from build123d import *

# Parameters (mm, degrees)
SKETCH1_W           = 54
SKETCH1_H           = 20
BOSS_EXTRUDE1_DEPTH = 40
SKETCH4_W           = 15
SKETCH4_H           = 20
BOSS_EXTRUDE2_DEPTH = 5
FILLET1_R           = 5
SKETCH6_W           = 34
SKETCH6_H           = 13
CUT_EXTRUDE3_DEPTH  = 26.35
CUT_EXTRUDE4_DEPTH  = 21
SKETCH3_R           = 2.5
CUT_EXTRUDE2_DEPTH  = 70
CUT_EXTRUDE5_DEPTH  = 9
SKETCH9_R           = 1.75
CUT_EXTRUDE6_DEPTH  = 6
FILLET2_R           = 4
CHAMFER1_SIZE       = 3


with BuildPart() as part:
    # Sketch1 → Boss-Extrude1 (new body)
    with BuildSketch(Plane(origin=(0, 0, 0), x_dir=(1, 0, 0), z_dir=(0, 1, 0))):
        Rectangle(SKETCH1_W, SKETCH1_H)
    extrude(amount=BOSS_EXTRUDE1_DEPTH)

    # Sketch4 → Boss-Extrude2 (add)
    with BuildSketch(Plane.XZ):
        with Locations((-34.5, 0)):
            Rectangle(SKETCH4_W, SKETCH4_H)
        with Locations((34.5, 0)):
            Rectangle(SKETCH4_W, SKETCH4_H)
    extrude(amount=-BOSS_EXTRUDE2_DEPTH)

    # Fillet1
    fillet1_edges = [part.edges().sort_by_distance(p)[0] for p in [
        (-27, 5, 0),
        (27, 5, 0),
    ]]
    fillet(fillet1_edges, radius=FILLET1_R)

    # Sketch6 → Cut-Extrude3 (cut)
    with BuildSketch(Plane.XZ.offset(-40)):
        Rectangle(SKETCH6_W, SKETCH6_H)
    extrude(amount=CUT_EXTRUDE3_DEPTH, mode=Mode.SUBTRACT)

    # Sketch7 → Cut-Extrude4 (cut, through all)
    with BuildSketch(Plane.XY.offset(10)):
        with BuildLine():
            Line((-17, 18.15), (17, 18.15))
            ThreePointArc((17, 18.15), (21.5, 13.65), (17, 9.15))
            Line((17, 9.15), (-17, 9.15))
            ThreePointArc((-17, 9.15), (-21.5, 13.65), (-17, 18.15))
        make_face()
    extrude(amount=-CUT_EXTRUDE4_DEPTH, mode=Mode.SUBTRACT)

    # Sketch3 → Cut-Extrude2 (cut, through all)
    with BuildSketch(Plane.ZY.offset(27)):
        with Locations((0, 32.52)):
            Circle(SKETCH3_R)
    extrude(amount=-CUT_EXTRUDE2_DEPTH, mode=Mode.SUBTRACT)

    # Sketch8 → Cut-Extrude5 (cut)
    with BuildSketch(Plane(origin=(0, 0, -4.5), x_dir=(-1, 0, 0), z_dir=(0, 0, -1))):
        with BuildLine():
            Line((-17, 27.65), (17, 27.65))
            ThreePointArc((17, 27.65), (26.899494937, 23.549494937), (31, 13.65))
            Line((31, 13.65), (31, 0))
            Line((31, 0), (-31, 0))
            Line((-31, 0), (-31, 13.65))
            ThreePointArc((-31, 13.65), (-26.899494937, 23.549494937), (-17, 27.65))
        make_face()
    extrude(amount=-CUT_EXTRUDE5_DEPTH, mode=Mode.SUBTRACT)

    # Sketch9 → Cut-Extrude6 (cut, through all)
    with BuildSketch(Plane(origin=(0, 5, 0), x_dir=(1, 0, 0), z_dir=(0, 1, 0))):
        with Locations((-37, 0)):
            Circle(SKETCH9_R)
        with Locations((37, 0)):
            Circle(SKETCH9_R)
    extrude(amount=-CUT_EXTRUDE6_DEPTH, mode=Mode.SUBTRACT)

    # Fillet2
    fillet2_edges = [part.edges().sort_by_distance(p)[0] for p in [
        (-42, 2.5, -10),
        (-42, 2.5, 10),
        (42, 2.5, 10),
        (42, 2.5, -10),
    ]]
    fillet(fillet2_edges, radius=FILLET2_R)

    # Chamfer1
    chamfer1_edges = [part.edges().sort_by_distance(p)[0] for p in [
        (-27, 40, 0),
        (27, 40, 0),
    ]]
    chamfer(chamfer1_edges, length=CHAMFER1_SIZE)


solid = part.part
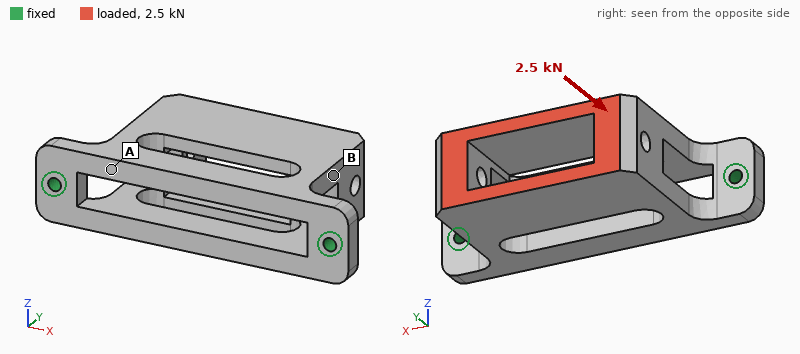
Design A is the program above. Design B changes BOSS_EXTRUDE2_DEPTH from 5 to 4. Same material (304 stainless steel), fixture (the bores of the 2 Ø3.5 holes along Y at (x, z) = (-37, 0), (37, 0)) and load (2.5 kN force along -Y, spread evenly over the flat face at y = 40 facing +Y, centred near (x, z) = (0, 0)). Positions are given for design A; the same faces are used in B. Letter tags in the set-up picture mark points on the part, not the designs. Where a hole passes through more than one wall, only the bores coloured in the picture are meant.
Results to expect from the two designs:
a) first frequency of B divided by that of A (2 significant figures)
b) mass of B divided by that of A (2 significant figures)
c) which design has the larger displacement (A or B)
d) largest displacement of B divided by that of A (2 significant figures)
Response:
0.80
0.98
B
1.3
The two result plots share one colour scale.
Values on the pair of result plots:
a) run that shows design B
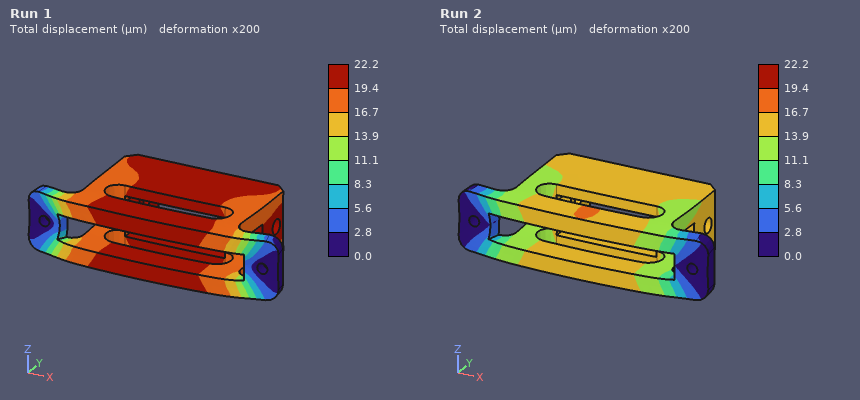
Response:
Run 1
